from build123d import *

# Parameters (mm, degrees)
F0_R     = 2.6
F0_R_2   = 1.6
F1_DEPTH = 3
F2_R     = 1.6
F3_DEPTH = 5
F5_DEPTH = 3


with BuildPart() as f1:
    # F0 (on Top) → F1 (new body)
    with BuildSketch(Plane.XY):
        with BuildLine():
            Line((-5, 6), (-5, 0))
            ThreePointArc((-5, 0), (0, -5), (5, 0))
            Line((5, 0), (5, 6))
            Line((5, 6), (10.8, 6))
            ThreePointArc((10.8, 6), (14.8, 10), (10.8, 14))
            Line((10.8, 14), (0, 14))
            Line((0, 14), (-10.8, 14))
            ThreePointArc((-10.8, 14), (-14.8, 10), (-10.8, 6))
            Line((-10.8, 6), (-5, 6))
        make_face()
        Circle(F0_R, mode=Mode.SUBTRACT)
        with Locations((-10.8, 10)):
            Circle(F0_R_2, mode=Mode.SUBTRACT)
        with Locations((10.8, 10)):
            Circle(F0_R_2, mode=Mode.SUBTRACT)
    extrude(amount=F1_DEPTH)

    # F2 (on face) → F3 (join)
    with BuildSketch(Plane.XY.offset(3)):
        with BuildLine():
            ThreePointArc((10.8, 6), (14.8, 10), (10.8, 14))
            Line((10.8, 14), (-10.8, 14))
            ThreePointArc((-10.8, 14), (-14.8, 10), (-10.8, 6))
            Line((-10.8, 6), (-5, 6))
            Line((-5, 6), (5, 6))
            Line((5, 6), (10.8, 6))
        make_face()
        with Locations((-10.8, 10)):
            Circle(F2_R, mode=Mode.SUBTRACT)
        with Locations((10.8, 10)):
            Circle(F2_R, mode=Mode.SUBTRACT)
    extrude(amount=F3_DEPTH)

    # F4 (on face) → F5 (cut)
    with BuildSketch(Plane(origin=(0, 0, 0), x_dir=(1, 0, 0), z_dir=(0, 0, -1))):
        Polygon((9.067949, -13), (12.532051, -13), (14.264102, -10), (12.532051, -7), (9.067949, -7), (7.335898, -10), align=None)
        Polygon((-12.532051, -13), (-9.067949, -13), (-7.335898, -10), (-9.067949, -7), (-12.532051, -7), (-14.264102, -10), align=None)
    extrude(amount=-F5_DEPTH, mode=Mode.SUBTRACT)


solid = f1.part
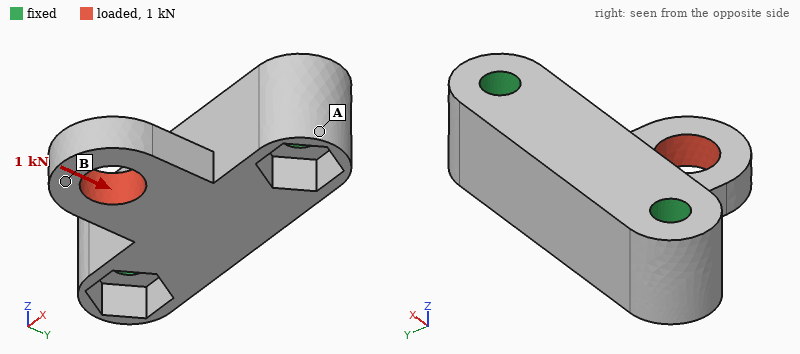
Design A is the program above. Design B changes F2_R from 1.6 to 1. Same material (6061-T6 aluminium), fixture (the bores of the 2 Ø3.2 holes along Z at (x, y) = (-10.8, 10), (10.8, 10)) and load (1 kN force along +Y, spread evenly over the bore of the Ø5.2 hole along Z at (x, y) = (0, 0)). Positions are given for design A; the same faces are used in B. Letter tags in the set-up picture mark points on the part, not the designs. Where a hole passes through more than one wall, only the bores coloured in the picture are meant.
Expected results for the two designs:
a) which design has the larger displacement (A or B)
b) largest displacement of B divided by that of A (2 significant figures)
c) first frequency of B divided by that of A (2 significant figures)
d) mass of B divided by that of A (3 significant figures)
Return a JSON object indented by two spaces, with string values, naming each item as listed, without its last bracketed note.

{
  "which design has the larger displacement": "B",
  "largest displacement of B divided by that of A": "1.2",
  "first frequency of B divided by that of A": "0.96",
  "mass of B divided by that of A": "1.03"
}
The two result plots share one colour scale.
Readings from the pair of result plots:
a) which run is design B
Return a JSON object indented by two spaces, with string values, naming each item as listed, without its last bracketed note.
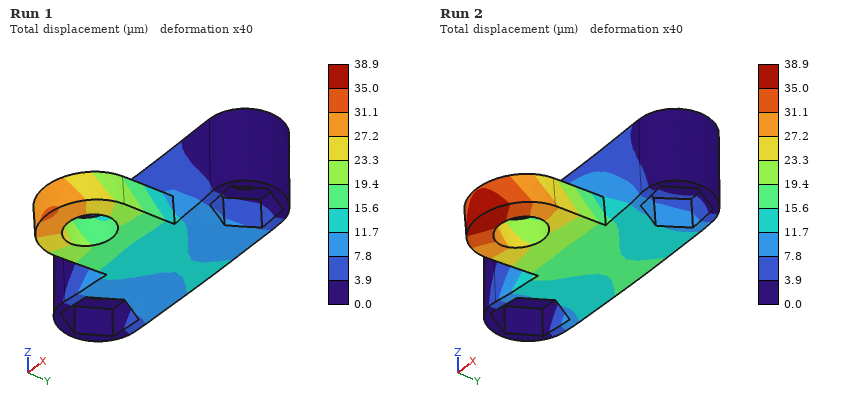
{
  "which run is design B": "Run 2"
}
